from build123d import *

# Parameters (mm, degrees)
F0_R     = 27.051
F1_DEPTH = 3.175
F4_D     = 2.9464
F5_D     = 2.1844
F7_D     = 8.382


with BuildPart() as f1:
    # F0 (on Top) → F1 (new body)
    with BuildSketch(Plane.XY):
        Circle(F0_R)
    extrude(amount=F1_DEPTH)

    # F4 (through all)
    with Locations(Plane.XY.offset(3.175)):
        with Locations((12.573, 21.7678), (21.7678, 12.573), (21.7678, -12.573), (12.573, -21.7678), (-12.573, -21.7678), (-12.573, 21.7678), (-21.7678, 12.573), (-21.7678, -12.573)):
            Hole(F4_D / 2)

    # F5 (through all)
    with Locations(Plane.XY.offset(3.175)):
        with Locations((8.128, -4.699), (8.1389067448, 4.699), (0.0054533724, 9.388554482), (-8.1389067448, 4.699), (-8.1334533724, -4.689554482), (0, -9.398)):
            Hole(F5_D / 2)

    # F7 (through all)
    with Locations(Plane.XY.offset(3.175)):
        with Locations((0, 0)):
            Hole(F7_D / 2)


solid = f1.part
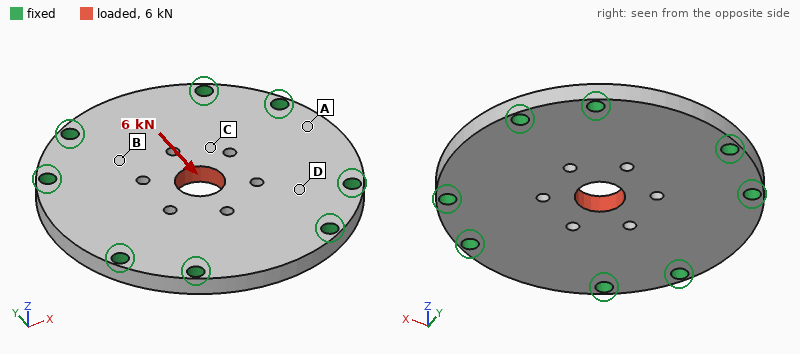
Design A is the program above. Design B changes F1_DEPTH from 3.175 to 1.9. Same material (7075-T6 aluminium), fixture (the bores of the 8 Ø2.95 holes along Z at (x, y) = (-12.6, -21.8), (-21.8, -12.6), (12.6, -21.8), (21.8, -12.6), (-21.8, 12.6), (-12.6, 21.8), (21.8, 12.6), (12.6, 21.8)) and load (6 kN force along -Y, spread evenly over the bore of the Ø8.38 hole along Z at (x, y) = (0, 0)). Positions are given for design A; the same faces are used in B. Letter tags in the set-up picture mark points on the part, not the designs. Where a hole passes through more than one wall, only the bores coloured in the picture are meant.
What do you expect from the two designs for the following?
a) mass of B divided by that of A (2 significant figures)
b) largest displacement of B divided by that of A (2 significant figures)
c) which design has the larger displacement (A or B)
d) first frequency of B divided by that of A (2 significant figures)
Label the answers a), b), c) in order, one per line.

a) 0.60
b) 1.7
c) B
d) 0.64
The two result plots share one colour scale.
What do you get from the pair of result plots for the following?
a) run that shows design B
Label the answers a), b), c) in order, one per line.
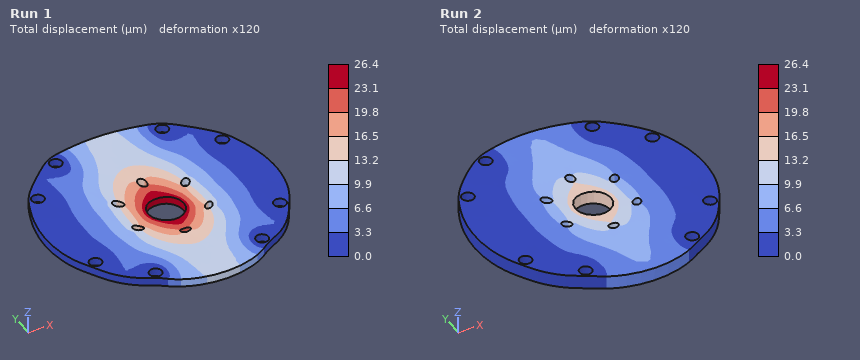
a) Run 1
